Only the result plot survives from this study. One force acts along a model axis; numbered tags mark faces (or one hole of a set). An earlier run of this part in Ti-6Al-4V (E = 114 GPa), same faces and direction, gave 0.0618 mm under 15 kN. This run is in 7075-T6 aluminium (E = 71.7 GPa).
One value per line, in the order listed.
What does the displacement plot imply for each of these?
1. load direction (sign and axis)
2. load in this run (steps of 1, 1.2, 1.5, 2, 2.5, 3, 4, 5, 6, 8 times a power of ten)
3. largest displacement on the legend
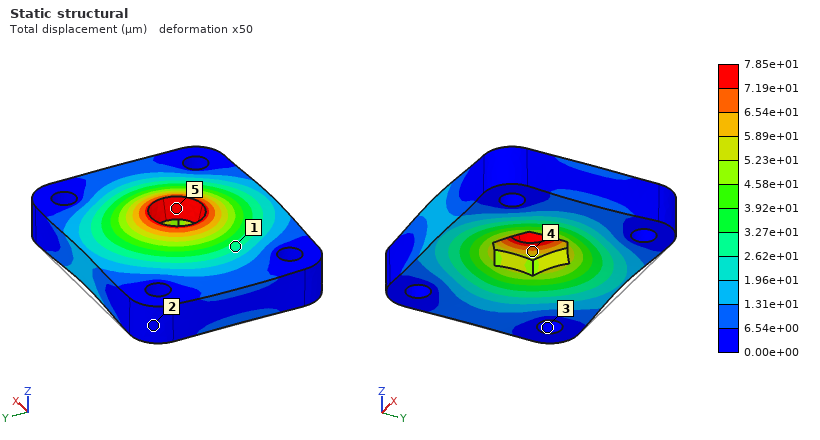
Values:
+Z
12 kN
7.85e+01 µm
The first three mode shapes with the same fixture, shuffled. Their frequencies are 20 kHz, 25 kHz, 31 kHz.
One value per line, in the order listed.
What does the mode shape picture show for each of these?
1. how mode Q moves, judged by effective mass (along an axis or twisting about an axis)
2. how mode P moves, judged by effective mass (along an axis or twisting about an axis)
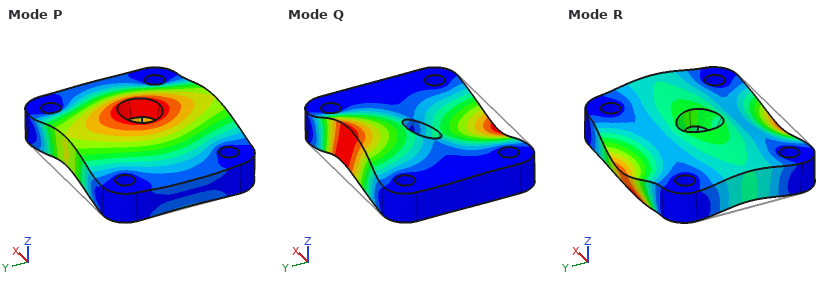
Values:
twisting about X
along Z
